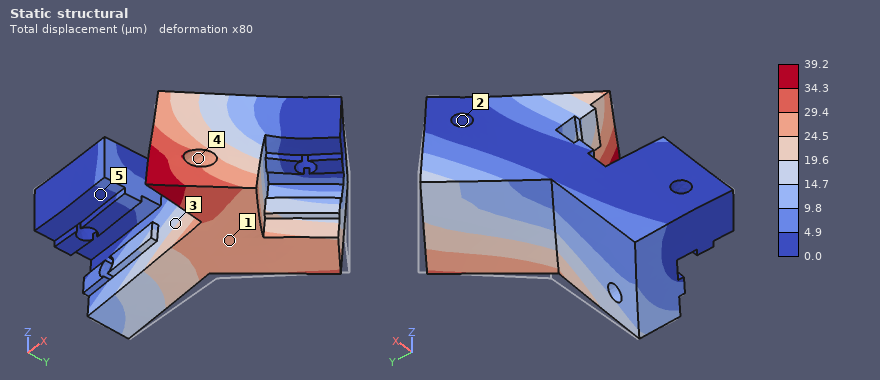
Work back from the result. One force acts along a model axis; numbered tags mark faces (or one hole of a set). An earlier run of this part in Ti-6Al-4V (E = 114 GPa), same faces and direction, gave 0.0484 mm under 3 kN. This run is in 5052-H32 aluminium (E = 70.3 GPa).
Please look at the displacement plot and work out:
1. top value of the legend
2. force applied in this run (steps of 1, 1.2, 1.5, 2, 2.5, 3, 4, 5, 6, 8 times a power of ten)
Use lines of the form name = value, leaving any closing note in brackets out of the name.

top value of the legend = 39.2 µm
force applied in this run = 1.5 kN
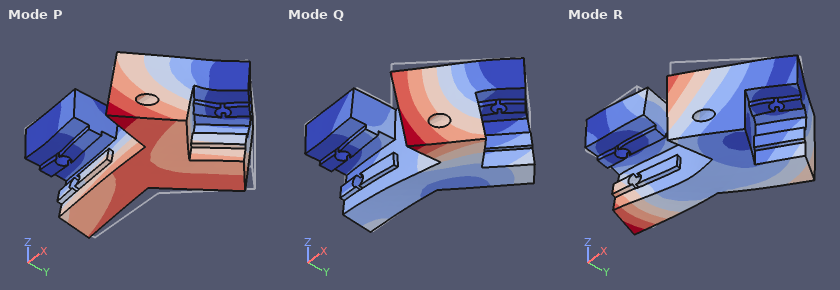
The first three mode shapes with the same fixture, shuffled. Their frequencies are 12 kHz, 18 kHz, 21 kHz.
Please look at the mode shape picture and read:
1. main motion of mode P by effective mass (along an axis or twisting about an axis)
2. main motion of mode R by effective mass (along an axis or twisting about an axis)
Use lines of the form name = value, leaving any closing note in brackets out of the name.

main motion of mode P by effective mass = along Y
main motion of mode R by effective mass = along Z
